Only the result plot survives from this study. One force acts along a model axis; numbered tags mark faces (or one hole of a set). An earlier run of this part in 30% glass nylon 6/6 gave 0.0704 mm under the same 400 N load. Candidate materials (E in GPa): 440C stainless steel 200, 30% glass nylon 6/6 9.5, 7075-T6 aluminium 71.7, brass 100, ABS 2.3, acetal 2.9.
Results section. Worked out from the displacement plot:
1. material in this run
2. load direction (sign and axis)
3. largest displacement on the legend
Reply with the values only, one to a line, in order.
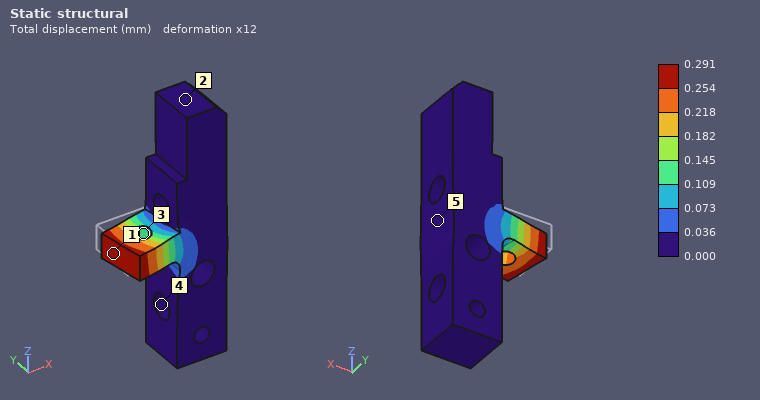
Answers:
ABS
-Y
0.291 mm
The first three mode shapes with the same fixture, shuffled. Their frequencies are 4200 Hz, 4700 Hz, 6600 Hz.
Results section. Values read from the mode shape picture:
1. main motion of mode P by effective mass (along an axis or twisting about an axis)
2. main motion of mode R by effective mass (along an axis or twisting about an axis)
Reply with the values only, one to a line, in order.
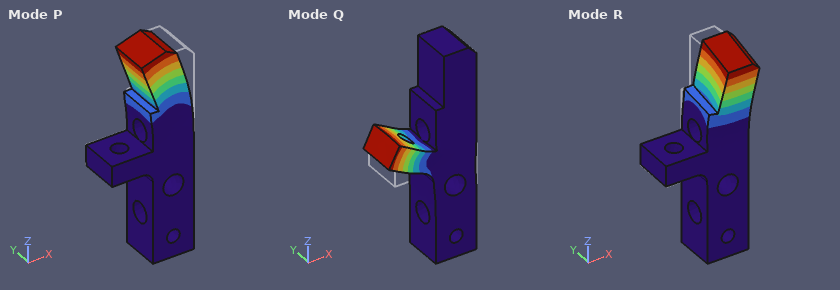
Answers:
along X
along Y
